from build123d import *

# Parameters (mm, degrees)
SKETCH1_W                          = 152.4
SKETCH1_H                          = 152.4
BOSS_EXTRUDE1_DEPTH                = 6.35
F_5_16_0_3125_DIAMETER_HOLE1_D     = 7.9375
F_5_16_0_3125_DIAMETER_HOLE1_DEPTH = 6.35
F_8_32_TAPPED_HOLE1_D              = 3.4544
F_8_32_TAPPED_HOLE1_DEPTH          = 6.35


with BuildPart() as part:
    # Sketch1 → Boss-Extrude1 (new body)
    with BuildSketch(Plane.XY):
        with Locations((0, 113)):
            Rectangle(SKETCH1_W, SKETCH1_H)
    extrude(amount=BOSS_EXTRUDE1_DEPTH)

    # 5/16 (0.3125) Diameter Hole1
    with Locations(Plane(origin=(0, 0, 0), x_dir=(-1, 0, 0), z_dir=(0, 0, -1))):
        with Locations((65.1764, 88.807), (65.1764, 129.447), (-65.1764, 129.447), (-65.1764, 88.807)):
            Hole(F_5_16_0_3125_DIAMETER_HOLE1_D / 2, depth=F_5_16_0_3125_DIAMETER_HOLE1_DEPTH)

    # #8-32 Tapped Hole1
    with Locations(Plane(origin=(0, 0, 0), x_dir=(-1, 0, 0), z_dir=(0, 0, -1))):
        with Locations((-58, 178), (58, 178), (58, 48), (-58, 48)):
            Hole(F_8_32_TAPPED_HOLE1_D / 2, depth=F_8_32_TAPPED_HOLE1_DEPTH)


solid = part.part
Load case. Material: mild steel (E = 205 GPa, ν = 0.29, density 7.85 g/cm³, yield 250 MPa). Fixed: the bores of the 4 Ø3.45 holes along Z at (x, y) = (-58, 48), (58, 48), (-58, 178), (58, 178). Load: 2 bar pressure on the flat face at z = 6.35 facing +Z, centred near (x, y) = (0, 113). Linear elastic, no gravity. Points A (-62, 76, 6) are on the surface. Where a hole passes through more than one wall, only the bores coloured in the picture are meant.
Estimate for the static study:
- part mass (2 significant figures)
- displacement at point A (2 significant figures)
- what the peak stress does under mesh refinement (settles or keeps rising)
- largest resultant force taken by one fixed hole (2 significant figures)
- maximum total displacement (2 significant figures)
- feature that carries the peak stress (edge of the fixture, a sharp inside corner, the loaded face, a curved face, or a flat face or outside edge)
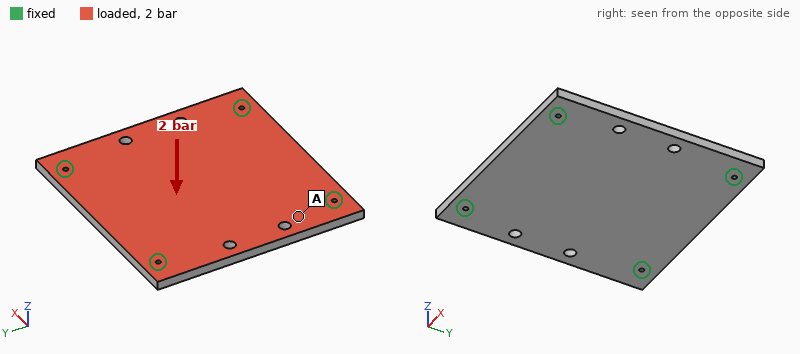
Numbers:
1.1 kg
32 µm
keeps rising
1.2 kN
91 µm
edge of the fixture
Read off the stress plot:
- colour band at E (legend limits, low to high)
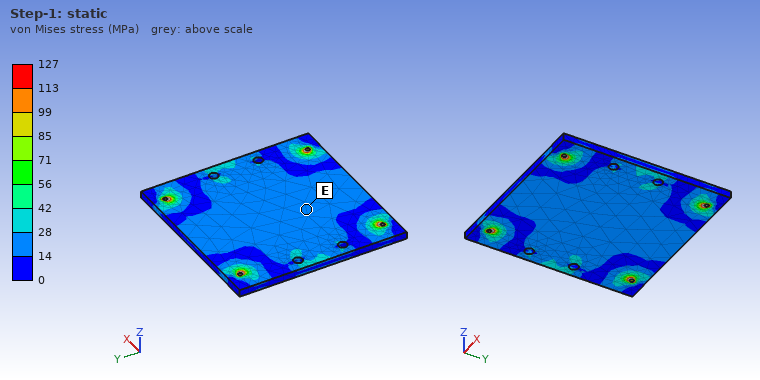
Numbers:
14 to 28 MPa
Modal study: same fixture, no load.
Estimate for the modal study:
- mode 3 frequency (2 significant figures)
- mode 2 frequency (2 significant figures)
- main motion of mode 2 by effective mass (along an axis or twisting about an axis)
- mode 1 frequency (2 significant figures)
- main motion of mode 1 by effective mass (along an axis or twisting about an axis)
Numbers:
2300 Hz
2000 Hz
twisting about Y
1300 Hz
along Z
